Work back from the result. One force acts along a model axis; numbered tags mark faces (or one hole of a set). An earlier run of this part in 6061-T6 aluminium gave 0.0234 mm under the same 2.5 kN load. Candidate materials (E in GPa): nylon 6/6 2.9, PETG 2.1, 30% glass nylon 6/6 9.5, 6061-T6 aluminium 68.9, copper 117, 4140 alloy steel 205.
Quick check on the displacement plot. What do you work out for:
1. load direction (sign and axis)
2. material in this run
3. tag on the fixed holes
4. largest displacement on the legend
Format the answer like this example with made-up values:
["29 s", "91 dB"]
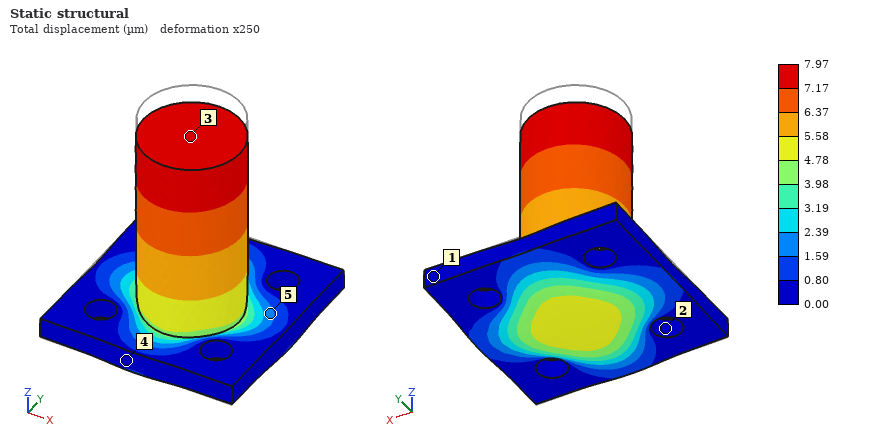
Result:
["-Z", "4140 alloy steel", "2", "7.97 µm"]
